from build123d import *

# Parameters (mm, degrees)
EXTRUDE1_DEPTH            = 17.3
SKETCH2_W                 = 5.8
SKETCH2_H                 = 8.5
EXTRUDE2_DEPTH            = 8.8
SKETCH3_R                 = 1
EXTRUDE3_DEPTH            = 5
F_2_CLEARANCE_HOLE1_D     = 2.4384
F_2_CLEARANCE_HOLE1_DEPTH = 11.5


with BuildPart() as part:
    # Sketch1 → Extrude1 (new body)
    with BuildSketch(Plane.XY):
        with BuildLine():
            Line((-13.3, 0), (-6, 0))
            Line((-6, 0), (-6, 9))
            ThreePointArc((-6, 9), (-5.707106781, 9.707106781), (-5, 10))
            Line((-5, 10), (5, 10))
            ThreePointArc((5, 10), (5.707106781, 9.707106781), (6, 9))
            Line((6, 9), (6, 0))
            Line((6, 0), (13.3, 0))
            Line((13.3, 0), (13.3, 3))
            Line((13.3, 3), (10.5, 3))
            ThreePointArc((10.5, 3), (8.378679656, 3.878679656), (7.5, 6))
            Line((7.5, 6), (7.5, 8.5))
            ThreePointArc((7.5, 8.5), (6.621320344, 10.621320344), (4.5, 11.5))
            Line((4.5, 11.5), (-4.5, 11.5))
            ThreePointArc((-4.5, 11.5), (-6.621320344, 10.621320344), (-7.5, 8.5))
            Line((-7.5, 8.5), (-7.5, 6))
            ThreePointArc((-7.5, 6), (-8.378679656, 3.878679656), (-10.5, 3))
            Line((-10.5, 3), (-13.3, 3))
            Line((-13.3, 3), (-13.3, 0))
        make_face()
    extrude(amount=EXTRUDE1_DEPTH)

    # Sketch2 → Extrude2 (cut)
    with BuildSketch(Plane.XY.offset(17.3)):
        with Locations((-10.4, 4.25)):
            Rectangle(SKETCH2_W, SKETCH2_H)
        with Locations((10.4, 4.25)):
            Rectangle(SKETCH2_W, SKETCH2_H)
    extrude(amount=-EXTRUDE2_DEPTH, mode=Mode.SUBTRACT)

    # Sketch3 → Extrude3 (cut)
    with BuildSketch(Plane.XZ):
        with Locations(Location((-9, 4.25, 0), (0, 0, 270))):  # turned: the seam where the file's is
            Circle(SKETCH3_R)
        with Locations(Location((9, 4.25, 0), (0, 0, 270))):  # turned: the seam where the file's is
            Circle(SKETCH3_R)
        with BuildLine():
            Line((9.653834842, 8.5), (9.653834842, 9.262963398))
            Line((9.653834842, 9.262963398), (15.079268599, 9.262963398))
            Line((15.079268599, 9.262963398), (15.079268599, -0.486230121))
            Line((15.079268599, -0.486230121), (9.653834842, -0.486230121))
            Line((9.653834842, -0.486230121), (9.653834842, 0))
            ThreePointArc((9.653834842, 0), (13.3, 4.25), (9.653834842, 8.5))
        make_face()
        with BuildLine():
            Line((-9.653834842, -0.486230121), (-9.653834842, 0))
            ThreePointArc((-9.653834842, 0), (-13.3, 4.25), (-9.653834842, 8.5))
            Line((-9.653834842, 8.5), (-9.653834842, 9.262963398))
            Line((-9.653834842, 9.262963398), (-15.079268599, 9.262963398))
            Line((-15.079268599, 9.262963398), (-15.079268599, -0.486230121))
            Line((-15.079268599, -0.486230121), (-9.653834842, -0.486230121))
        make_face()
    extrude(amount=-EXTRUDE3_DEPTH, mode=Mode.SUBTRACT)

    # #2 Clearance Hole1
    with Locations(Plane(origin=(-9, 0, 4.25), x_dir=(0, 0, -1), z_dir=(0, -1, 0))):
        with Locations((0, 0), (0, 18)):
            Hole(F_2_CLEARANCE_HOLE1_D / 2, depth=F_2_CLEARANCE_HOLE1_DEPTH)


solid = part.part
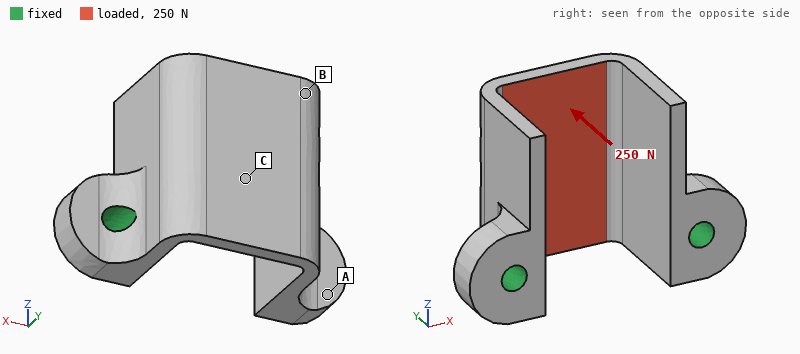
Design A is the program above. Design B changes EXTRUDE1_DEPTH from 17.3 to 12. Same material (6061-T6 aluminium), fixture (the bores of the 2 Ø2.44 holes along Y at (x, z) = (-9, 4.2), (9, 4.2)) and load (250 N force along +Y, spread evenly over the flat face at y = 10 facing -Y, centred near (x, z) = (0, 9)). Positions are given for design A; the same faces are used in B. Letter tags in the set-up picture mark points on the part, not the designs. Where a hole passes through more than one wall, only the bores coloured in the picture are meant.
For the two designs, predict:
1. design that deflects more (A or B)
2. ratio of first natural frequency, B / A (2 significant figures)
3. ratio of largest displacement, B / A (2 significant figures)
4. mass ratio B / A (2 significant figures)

A
1.3
0.82
0.76
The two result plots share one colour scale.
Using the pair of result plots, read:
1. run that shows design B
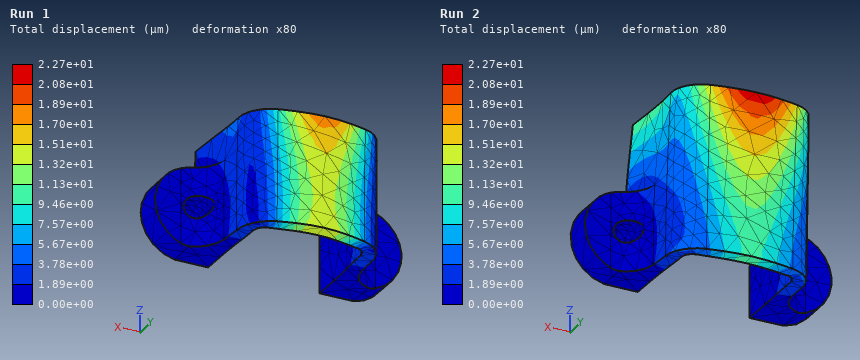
Run 1
